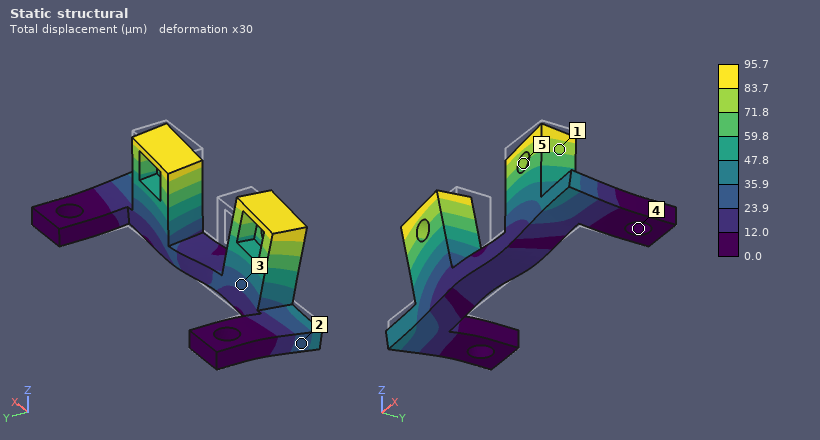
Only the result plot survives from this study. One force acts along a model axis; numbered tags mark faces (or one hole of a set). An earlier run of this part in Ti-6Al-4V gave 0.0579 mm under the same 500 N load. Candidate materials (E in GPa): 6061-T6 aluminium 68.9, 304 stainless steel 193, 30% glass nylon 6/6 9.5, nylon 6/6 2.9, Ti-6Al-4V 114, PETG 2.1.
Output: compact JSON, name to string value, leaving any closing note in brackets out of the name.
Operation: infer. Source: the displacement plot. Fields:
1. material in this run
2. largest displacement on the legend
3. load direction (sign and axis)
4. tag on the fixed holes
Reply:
{"material in this run": "6061-T6 aluminium", "largest displacement on the legend": "95.7 µm", "load direction": "-X", "tag on the fixed holes": "4"}
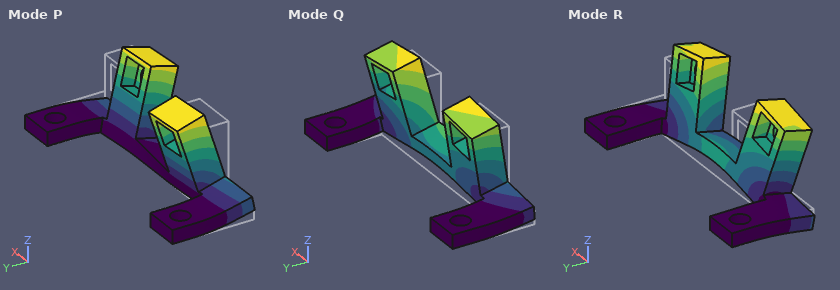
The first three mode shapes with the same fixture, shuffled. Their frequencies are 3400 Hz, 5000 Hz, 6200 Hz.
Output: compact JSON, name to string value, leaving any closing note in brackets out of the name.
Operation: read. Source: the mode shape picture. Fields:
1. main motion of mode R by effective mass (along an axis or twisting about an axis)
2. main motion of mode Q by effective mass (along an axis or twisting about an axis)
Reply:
{"main motion of mode R by effective mass": "along Y", "main motion of mode Q by effective mass": "along Z"}
